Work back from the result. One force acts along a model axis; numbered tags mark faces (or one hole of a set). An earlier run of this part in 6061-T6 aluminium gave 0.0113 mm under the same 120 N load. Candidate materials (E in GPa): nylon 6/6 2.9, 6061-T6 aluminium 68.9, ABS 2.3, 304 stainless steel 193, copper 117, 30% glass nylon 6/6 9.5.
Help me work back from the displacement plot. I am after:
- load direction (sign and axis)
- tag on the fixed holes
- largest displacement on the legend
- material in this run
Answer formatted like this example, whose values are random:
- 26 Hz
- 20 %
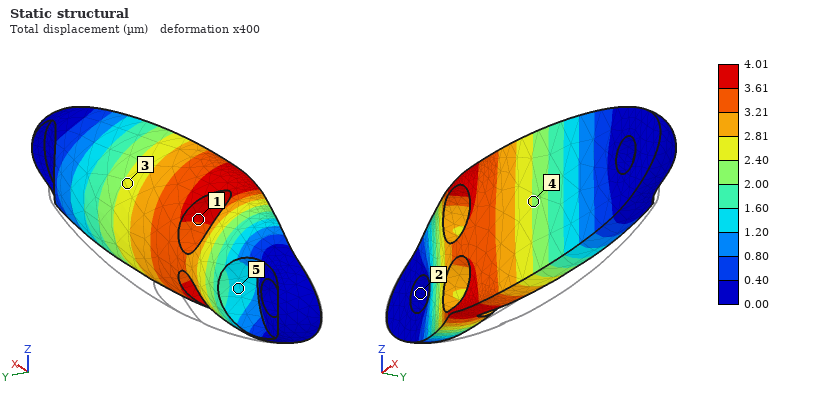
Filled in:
- -Y
- 2
- 4.01 µm
- 304 stainless steel
